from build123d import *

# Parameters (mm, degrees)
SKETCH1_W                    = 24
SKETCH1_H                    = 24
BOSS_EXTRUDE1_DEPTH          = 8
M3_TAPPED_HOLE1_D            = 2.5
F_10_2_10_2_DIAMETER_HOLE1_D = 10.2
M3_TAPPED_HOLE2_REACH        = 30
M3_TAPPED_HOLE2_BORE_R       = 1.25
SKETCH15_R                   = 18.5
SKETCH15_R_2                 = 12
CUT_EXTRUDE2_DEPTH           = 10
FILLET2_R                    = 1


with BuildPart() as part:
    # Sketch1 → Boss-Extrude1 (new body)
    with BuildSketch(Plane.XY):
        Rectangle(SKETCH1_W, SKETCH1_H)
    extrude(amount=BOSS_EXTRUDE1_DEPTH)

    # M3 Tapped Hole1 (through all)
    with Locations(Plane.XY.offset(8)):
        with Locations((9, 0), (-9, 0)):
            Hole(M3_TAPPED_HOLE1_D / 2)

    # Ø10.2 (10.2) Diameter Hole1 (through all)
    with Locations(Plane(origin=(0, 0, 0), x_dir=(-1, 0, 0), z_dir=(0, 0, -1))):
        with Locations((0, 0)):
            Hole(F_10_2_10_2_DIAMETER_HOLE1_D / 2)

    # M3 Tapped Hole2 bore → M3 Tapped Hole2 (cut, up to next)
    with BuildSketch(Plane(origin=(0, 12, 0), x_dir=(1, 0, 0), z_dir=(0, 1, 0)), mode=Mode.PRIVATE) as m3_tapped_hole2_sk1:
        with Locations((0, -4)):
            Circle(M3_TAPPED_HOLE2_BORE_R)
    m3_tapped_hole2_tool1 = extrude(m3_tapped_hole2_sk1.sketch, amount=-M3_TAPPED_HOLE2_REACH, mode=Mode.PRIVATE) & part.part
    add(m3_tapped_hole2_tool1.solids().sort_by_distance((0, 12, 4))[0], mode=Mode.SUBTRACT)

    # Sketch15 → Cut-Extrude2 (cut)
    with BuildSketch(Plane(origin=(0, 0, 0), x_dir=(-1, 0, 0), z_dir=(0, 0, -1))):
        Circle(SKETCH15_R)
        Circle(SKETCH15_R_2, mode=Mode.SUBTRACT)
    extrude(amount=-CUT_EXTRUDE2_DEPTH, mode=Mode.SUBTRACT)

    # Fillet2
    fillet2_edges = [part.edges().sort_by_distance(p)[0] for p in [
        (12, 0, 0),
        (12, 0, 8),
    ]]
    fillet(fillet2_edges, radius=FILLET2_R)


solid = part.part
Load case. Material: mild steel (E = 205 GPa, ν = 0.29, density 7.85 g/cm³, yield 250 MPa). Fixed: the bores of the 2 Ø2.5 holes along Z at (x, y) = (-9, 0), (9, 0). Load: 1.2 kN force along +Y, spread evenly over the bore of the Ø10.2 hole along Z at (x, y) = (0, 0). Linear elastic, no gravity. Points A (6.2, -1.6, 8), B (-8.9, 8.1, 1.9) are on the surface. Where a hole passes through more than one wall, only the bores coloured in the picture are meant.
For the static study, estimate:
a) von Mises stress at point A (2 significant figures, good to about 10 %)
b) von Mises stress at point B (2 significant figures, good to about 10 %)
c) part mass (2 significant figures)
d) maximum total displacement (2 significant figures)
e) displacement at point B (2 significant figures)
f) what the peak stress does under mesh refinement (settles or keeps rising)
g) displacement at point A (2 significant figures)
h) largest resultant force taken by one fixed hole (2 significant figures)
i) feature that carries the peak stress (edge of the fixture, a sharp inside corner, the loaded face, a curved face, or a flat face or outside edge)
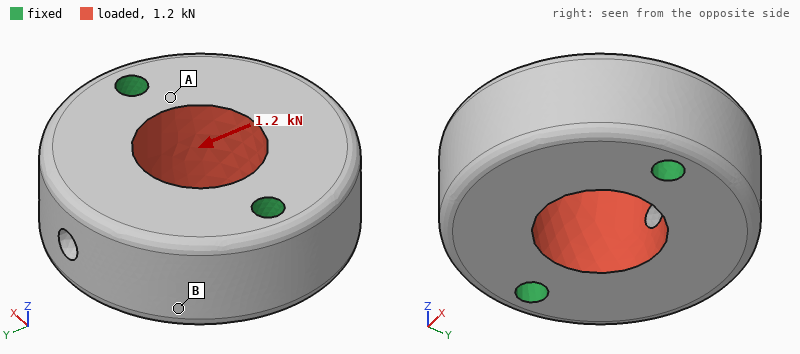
10 MPa
3.2 MPa
22 g
0.50 µm
0.18 µm
keeps rising
0.21 µm
600 N
edge of the fixture
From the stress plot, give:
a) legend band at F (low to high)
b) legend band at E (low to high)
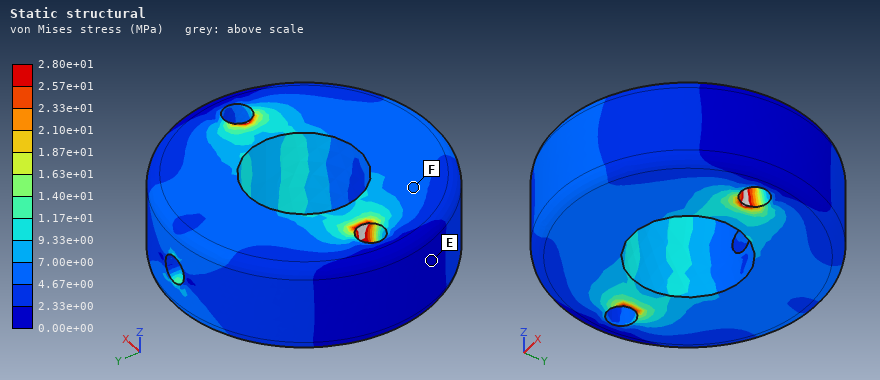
4.67e+00 to 7.00e+00 MPa
0.00e+00 to 2.33e+00 MPa
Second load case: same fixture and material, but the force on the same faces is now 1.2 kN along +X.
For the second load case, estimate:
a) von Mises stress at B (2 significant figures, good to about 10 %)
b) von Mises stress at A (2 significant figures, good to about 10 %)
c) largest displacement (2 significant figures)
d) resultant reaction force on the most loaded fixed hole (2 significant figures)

2.6 MPa
12 MPa
0.52 µm
600 N
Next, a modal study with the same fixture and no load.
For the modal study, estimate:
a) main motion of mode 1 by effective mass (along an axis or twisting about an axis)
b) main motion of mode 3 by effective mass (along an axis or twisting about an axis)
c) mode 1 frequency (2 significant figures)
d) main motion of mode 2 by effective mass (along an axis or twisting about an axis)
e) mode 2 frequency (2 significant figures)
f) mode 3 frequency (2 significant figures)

twisting about X
twisting about Z
32 kHz
along Z
36 kHz
51 kHz
